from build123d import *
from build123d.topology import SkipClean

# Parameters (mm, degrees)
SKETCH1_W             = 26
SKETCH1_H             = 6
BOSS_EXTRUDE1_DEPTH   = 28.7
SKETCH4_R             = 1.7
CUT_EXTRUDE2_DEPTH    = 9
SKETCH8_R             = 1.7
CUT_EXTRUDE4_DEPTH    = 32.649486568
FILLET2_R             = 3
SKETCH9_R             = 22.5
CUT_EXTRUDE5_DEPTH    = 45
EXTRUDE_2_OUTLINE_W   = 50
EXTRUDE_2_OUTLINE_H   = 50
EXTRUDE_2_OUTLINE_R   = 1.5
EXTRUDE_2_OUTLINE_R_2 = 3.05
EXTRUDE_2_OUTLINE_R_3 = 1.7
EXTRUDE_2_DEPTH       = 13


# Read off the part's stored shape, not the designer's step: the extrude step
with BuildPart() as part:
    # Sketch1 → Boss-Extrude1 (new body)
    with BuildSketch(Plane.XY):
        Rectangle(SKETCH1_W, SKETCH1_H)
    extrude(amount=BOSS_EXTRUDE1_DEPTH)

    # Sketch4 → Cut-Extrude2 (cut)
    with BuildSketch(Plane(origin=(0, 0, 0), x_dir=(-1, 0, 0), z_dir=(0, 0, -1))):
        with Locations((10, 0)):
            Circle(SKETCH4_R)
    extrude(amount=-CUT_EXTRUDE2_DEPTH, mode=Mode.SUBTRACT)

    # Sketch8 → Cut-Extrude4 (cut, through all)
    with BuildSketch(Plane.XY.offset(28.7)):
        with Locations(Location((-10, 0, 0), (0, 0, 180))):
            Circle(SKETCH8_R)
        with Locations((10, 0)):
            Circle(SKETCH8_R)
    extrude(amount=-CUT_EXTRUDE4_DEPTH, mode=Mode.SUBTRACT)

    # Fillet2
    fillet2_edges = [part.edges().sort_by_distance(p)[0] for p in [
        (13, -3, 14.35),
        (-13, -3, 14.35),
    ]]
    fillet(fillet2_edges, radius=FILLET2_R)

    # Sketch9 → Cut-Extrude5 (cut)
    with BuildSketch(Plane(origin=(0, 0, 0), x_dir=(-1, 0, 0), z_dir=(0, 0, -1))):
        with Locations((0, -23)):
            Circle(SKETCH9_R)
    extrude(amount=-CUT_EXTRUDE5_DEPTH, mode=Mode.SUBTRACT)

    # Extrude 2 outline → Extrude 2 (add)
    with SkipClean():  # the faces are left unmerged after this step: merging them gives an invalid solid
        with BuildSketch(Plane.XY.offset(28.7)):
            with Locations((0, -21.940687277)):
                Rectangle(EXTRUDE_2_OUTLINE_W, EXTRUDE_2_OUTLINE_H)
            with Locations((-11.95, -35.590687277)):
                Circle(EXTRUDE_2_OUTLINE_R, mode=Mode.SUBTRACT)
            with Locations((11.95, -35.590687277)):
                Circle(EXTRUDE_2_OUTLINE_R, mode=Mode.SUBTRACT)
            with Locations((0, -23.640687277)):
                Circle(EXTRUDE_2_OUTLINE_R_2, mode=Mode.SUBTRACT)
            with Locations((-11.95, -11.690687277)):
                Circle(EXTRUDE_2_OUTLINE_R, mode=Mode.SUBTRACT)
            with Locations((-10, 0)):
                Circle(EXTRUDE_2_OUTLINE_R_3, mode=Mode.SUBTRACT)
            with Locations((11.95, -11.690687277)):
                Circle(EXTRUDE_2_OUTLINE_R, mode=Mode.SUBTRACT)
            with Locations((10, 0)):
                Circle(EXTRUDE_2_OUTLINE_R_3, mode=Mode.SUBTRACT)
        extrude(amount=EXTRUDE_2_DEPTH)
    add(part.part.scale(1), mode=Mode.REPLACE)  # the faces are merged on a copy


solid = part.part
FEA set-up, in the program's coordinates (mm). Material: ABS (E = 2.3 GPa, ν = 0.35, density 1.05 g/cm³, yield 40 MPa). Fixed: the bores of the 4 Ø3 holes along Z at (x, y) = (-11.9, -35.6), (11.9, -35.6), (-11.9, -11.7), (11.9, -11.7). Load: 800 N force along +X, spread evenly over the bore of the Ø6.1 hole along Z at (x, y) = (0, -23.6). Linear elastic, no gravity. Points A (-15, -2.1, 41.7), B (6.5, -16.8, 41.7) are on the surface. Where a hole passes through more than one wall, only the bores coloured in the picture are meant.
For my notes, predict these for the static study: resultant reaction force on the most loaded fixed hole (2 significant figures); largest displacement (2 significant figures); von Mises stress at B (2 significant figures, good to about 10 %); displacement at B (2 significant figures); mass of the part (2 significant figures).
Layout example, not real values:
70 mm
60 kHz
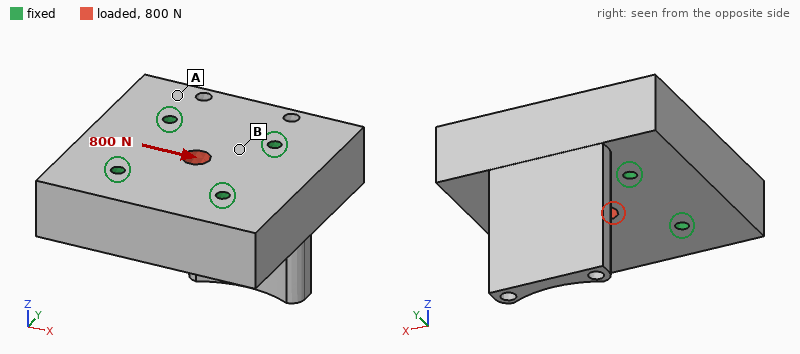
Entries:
210 N
16 µm
1.8 MPa
6.1 µm
36 g
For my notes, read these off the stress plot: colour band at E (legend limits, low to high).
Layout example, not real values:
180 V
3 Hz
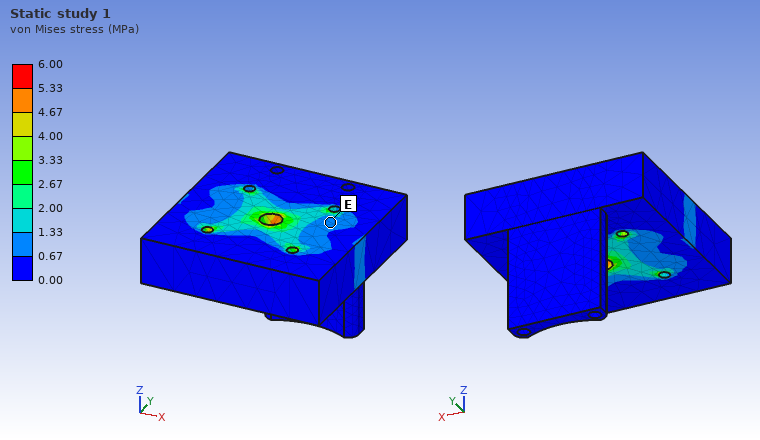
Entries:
0.67 to 1.33 MPa
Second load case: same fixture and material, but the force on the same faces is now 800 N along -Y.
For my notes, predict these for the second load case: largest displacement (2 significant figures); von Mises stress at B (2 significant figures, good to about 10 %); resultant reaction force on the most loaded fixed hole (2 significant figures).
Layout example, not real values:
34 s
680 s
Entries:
16 µm
1.8 MPa
210 N
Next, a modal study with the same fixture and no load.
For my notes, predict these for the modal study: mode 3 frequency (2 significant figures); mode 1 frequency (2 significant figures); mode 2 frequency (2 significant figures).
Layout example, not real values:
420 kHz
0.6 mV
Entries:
3600 Hz
1200 Hz
2900 Hz
